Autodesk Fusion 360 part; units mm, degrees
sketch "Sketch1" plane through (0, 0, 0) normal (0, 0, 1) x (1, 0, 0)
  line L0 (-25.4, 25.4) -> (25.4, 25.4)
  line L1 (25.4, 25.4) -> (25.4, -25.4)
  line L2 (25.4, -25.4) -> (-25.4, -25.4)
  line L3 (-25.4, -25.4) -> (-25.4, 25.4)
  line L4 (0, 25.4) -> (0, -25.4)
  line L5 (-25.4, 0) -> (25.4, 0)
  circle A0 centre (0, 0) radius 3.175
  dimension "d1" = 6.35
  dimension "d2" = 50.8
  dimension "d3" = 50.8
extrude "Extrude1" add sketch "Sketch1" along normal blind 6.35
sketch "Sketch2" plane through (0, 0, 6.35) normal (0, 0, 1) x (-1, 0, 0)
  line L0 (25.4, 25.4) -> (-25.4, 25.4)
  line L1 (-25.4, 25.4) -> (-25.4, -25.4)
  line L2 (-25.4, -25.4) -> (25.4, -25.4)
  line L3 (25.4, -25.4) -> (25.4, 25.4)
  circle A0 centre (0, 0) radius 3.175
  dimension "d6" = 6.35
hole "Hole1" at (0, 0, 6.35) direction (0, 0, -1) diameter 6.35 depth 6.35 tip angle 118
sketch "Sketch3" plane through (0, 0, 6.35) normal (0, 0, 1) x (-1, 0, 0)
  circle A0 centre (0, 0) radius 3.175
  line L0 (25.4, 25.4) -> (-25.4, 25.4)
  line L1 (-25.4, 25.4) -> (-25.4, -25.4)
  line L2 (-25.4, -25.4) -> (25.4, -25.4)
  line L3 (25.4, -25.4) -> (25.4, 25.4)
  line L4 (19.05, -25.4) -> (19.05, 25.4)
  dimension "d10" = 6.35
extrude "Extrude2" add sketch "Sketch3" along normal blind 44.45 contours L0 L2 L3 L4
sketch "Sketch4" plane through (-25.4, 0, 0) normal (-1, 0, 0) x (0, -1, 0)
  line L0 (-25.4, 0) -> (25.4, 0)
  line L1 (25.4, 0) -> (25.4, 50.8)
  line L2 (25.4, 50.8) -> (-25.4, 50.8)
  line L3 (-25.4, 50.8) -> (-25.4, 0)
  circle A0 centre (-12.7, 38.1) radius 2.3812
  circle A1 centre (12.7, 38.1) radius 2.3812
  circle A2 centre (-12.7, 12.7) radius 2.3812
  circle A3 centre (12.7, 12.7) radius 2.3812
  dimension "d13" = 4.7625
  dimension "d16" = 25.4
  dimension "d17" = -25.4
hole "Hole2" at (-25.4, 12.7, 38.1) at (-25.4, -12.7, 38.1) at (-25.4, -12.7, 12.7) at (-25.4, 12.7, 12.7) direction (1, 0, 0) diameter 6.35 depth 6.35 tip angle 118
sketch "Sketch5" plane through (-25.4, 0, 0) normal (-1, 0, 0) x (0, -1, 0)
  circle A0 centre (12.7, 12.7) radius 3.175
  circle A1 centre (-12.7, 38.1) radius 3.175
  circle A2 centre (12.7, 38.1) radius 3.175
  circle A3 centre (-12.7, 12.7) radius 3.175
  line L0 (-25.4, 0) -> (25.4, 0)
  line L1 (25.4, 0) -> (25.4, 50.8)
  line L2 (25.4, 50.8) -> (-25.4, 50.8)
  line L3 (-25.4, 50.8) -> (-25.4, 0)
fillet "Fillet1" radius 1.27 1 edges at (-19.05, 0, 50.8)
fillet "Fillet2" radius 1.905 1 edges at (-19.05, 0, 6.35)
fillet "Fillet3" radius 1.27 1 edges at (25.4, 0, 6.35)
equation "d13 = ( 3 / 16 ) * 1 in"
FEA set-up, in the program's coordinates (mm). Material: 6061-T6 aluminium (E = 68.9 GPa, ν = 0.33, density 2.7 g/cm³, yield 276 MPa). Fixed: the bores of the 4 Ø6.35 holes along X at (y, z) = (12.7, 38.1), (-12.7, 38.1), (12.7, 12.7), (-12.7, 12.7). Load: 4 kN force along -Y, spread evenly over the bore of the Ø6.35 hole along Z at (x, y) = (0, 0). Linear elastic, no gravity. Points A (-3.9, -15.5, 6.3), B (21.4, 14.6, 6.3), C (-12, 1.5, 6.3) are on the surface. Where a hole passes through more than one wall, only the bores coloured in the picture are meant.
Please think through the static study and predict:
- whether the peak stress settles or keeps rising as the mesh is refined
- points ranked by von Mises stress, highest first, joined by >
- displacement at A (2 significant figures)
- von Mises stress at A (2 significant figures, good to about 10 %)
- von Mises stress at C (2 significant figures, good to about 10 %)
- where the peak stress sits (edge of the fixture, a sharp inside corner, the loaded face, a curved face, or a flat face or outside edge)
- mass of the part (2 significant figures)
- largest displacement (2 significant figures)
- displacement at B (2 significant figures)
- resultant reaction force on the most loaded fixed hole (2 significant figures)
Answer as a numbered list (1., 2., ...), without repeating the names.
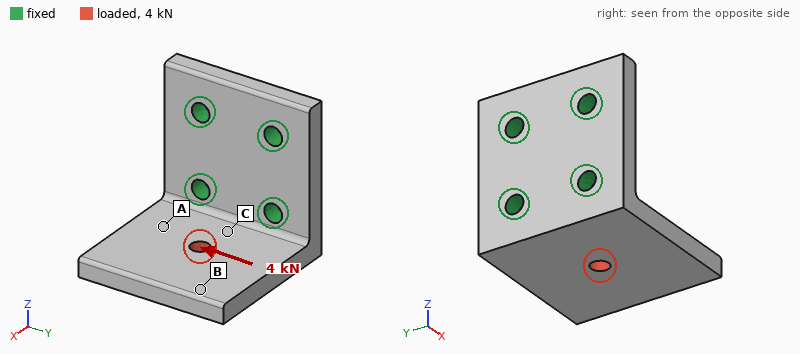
1. keeps rising
2. C > A > B
3. 48 µm
4. 30 MPa
5. 52 MPa
6. edge of the fixture
7. 80 g
8. 100 µm
9. 86 µm
10. 3.7 kN
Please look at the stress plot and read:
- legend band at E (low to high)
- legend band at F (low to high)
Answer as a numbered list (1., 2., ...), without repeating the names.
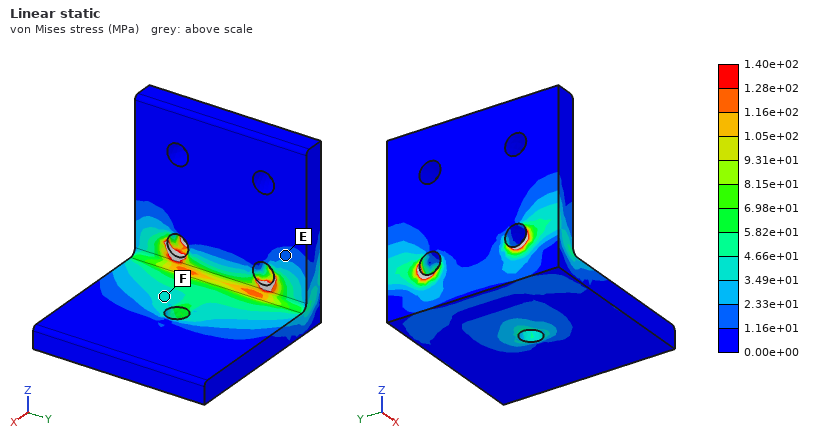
1. 1.16e+01 to 2.33e+01 MPa
2. 3.49e+01 to 4.66e+01 MPa
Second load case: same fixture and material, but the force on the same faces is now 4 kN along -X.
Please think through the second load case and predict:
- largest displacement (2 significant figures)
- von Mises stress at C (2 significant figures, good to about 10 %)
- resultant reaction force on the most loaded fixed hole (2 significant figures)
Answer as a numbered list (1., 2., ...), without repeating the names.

1. 0.11 mm
2. 18 MPa
3. 2.1 kN
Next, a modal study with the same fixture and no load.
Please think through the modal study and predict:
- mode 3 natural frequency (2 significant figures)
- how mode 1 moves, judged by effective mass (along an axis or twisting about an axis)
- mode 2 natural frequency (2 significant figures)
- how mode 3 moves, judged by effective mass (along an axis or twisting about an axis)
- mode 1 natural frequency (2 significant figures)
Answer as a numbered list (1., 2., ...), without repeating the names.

1. 6300 Hz
2. along Z
3. 4400 Hz
4. along Y
5. 1900 Hz
